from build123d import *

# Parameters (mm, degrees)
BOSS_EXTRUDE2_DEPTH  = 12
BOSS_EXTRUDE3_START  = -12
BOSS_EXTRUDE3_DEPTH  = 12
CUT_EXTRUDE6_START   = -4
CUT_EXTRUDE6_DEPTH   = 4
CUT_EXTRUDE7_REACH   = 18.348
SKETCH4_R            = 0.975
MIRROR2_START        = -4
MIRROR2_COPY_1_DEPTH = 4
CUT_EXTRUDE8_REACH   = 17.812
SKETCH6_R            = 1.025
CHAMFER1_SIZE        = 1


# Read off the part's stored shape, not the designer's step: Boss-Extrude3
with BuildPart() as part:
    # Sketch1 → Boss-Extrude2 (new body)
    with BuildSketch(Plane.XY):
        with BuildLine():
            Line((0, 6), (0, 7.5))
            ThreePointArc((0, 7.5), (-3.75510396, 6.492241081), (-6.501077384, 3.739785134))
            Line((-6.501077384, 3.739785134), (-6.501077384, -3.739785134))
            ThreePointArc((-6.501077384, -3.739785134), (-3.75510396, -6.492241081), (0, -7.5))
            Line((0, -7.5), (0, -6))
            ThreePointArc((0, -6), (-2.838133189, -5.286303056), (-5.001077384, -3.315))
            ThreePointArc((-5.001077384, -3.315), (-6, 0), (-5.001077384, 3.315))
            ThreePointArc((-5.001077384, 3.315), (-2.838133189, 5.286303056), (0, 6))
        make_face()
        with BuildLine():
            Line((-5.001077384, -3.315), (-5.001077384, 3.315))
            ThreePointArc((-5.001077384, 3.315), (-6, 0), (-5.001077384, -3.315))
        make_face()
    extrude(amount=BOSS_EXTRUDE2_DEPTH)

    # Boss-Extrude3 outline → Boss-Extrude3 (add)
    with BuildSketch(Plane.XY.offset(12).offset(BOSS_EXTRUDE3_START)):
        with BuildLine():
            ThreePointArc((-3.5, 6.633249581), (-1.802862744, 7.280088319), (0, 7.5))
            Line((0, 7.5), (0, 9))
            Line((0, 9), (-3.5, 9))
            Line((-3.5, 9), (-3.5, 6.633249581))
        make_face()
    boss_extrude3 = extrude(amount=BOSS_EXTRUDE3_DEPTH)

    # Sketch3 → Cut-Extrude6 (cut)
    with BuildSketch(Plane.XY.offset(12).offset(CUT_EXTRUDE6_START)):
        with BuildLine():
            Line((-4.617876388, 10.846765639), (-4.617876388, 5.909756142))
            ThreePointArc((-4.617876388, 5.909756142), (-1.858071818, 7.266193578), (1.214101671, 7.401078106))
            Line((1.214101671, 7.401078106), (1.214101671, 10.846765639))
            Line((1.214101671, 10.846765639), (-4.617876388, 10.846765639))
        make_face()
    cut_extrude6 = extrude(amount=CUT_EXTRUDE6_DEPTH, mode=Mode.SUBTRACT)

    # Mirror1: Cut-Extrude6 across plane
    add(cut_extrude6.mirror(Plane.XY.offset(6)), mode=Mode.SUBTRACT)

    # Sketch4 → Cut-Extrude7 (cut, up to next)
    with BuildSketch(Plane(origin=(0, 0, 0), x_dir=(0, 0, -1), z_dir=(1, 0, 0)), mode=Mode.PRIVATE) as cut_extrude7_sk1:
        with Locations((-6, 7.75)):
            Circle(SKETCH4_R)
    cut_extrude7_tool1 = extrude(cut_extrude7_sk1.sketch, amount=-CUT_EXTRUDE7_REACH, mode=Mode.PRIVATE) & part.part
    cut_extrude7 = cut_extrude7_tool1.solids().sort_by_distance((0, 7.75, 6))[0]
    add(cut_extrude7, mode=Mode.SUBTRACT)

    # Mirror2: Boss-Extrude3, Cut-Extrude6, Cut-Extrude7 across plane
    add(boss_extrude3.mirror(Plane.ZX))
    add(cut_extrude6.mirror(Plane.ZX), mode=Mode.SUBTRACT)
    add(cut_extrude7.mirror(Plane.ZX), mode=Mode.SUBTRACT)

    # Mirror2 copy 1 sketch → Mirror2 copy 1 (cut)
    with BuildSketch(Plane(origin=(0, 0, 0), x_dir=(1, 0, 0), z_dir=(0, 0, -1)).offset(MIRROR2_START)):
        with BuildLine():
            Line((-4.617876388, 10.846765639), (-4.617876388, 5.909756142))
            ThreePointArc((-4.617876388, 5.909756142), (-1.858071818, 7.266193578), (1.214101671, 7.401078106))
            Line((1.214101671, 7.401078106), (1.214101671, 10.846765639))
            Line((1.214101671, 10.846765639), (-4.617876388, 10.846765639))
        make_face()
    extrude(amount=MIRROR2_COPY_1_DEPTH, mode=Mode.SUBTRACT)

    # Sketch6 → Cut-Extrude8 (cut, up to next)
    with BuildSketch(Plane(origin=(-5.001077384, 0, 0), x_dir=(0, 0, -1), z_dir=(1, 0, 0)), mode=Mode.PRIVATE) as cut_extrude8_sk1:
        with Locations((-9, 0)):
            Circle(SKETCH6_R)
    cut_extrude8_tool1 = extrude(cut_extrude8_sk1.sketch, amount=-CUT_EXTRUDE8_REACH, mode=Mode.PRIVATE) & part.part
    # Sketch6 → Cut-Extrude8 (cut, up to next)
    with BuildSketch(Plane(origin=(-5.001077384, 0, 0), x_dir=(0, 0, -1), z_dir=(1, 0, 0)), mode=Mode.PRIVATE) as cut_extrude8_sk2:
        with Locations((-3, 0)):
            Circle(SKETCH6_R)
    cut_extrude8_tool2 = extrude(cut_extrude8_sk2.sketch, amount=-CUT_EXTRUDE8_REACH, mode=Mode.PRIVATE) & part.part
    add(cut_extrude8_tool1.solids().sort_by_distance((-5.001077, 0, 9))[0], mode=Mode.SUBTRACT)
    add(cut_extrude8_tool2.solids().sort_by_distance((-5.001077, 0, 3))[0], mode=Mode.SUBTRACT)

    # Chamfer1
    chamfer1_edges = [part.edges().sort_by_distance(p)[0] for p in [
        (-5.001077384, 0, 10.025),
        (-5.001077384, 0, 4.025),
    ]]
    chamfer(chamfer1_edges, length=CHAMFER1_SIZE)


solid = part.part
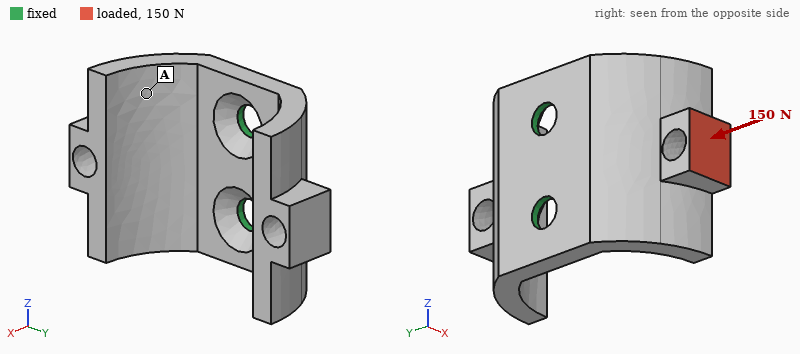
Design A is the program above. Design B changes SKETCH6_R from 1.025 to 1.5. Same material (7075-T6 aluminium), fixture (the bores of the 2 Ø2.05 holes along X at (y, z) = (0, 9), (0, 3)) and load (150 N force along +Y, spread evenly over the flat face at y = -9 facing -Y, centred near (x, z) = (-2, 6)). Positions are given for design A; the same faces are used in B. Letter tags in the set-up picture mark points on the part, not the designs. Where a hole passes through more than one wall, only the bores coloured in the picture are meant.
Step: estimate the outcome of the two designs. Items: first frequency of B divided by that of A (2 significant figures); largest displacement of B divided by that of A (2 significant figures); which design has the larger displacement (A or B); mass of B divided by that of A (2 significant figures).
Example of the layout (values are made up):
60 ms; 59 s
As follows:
1.2; 0.88; A; 0.96
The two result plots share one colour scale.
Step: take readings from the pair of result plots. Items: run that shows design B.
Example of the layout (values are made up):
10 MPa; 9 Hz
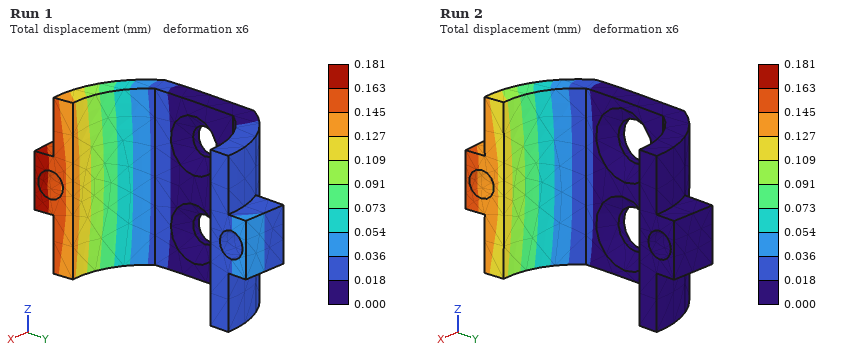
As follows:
Run 2
